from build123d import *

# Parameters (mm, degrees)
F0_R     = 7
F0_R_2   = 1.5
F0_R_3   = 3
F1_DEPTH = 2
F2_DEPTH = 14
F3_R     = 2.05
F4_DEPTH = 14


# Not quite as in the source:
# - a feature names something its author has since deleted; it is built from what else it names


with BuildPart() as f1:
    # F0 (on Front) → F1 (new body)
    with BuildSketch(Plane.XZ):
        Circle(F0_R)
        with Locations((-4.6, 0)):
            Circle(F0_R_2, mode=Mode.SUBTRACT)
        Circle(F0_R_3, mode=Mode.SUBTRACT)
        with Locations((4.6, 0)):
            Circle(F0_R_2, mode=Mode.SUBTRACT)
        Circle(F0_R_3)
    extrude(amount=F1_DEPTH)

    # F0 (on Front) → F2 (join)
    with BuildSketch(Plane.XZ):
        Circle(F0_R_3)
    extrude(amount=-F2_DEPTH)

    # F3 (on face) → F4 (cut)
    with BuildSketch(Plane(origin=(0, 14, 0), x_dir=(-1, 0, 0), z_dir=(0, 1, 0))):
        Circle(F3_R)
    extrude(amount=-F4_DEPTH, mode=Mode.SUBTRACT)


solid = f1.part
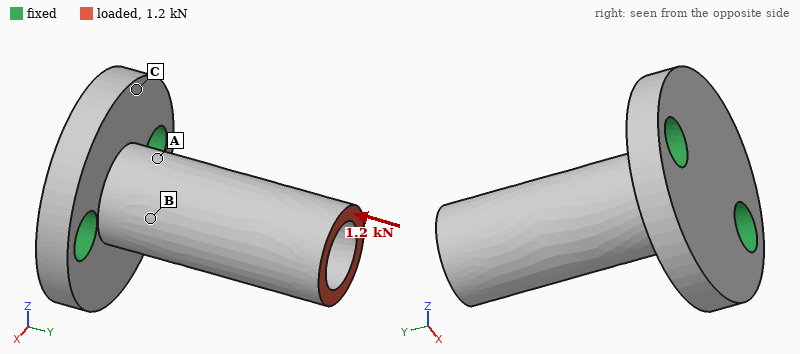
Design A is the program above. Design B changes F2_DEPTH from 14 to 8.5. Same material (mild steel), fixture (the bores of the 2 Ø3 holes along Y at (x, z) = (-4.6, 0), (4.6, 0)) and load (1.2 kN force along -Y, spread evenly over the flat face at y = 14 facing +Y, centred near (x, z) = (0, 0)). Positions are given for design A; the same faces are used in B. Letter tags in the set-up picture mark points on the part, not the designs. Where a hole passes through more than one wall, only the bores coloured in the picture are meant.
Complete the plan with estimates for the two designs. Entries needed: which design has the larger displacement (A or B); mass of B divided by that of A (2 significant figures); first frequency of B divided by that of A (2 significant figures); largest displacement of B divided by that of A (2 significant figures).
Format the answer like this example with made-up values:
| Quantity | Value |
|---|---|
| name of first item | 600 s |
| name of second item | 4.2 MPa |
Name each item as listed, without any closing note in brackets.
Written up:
| Quantity | Value |
|---|---|
| which design has the larger displacement | A |
| mass of B divided by that of A | 0.83 |
| first frequency of B divided by that of A | 1.9 |
| largest displacement of B divided by that of A | 0.69 |
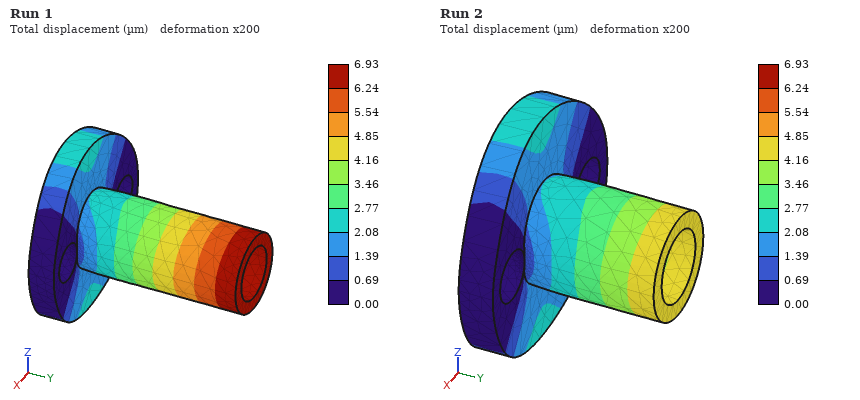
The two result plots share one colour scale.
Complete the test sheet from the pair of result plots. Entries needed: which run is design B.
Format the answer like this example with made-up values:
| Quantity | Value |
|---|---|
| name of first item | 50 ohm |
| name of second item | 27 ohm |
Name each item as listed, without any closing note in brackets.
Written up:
| Quantity | Value |
|---|---|
| which run is design B | Run 2 |
